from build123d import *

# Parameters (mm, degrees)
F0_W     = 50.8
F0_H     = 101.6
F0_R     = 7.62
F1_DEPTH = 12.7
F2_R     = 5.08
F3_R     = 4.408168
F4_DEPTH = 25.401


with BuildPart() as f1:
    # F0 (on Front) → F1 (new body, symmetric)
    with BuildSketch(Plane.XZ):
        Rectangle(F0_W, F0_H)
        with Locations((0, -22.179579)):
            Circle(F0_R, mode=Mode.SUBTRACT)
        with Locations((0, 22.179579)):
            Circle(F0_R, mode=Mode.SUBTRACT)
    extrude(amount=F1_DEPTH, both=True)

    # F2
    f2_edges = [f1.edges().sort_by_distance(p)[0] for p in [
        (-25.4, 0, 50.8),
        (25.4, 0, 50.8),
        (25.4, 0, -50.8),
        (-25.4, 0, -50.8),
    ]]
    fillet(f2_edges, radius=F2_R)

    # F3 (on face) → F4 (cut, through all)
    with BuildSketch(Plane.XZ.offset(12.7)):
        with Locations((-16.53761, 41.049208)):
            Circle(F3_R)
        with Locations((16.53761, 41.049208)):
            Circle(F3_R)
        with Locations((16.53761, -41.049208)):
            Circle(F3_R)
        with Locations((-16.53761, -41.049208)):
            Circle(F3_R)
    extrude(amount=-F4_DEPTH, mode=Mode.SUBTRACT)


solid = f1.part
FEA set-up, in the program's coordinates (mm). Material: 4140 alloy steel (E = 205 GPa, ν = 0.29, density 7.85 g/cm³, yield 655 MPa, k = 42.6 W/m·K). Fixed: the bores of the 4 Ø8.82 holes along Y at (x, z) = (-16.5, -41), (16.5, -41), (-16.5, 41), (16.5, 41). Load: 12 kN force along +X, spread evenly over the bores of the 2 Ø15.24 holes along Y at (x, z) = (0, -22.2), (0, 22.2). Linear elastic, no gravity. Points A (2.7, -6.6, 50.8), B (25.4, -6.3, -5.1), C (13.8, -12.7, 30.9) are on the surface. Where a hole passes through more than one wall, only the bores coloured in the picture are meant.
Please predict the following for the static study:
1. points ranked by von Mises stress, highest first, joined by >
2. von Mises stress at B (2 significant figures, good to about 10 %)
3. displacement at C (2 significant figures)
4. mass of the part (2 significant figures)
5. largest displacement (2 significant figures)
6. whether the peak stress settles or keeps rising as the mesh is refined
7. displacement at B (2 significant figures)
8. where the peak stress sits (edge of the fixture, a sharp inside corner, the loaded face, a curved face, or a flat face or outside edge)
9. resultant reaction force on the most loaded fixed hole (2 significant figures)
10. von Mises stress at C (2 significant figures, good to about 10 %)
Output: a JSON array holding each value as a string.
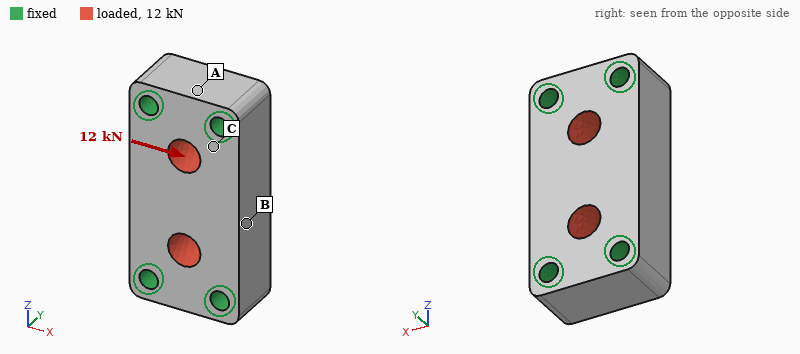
["C > B > A", "5.6 MPa", "0.62 µm", "900 g", "2.3 µm", "keeps rising", "2.2 µm", "edge of the fixture", "3.5 kN", "8.9 MPa"]
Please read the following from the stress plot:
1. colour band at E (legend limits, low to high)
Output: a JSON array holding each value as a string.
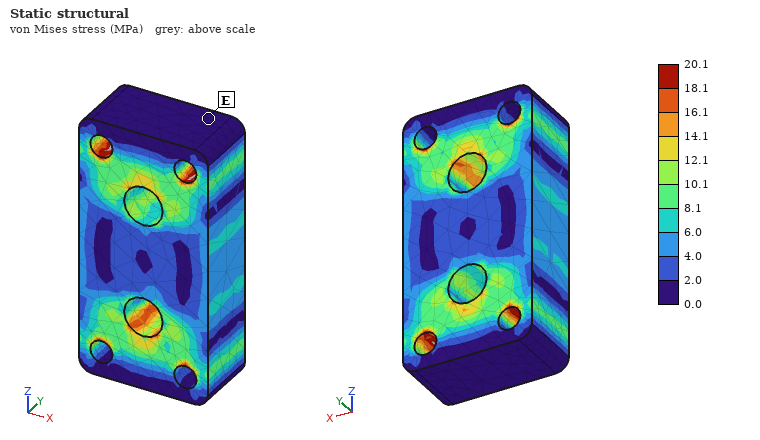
["0.0 to 2.0 MPa"]
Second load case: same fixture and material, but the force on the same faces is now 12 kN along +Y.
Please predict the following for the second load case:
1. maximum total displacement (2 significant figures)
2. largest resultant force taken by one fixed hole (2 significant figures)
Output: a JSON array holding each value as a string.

["3.1 µm", "3.0 kN"]
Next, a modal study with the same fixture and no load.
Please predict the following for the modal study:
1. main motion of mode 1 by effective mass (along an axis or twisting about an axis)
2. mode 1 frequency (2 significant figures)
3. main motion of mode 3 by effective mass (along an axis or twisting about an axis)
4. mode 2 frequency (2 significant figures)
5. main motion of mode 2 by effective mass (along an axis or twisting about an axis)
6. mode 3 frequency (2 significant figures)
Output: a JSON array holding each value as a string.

["along Y", "13 kHz", "twisting about Z", "14 kHz", "along X", "16 kHz"]
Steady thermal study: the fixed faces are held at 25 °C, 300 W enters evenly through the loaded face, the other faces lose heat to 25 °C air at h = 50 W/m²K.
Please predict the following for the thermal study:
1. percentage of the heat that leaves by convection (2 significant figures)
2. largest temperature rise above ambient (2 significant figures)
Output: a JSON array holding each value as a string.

["7.2 %", "71 K"]
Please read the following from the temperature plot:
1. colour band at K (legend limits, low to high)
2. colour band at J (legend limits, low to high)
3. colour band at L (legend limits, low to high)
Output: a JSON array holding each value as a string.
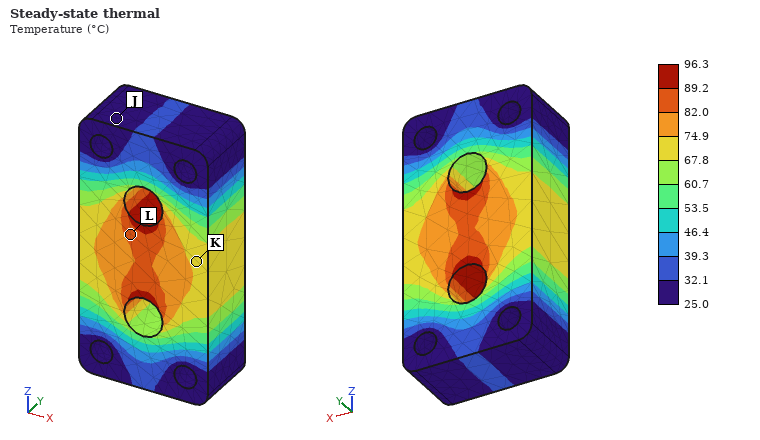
["67.8 to 74.9 °C", "25.0 to 32.1 °C", "82.0 to 89.2 °C"]
